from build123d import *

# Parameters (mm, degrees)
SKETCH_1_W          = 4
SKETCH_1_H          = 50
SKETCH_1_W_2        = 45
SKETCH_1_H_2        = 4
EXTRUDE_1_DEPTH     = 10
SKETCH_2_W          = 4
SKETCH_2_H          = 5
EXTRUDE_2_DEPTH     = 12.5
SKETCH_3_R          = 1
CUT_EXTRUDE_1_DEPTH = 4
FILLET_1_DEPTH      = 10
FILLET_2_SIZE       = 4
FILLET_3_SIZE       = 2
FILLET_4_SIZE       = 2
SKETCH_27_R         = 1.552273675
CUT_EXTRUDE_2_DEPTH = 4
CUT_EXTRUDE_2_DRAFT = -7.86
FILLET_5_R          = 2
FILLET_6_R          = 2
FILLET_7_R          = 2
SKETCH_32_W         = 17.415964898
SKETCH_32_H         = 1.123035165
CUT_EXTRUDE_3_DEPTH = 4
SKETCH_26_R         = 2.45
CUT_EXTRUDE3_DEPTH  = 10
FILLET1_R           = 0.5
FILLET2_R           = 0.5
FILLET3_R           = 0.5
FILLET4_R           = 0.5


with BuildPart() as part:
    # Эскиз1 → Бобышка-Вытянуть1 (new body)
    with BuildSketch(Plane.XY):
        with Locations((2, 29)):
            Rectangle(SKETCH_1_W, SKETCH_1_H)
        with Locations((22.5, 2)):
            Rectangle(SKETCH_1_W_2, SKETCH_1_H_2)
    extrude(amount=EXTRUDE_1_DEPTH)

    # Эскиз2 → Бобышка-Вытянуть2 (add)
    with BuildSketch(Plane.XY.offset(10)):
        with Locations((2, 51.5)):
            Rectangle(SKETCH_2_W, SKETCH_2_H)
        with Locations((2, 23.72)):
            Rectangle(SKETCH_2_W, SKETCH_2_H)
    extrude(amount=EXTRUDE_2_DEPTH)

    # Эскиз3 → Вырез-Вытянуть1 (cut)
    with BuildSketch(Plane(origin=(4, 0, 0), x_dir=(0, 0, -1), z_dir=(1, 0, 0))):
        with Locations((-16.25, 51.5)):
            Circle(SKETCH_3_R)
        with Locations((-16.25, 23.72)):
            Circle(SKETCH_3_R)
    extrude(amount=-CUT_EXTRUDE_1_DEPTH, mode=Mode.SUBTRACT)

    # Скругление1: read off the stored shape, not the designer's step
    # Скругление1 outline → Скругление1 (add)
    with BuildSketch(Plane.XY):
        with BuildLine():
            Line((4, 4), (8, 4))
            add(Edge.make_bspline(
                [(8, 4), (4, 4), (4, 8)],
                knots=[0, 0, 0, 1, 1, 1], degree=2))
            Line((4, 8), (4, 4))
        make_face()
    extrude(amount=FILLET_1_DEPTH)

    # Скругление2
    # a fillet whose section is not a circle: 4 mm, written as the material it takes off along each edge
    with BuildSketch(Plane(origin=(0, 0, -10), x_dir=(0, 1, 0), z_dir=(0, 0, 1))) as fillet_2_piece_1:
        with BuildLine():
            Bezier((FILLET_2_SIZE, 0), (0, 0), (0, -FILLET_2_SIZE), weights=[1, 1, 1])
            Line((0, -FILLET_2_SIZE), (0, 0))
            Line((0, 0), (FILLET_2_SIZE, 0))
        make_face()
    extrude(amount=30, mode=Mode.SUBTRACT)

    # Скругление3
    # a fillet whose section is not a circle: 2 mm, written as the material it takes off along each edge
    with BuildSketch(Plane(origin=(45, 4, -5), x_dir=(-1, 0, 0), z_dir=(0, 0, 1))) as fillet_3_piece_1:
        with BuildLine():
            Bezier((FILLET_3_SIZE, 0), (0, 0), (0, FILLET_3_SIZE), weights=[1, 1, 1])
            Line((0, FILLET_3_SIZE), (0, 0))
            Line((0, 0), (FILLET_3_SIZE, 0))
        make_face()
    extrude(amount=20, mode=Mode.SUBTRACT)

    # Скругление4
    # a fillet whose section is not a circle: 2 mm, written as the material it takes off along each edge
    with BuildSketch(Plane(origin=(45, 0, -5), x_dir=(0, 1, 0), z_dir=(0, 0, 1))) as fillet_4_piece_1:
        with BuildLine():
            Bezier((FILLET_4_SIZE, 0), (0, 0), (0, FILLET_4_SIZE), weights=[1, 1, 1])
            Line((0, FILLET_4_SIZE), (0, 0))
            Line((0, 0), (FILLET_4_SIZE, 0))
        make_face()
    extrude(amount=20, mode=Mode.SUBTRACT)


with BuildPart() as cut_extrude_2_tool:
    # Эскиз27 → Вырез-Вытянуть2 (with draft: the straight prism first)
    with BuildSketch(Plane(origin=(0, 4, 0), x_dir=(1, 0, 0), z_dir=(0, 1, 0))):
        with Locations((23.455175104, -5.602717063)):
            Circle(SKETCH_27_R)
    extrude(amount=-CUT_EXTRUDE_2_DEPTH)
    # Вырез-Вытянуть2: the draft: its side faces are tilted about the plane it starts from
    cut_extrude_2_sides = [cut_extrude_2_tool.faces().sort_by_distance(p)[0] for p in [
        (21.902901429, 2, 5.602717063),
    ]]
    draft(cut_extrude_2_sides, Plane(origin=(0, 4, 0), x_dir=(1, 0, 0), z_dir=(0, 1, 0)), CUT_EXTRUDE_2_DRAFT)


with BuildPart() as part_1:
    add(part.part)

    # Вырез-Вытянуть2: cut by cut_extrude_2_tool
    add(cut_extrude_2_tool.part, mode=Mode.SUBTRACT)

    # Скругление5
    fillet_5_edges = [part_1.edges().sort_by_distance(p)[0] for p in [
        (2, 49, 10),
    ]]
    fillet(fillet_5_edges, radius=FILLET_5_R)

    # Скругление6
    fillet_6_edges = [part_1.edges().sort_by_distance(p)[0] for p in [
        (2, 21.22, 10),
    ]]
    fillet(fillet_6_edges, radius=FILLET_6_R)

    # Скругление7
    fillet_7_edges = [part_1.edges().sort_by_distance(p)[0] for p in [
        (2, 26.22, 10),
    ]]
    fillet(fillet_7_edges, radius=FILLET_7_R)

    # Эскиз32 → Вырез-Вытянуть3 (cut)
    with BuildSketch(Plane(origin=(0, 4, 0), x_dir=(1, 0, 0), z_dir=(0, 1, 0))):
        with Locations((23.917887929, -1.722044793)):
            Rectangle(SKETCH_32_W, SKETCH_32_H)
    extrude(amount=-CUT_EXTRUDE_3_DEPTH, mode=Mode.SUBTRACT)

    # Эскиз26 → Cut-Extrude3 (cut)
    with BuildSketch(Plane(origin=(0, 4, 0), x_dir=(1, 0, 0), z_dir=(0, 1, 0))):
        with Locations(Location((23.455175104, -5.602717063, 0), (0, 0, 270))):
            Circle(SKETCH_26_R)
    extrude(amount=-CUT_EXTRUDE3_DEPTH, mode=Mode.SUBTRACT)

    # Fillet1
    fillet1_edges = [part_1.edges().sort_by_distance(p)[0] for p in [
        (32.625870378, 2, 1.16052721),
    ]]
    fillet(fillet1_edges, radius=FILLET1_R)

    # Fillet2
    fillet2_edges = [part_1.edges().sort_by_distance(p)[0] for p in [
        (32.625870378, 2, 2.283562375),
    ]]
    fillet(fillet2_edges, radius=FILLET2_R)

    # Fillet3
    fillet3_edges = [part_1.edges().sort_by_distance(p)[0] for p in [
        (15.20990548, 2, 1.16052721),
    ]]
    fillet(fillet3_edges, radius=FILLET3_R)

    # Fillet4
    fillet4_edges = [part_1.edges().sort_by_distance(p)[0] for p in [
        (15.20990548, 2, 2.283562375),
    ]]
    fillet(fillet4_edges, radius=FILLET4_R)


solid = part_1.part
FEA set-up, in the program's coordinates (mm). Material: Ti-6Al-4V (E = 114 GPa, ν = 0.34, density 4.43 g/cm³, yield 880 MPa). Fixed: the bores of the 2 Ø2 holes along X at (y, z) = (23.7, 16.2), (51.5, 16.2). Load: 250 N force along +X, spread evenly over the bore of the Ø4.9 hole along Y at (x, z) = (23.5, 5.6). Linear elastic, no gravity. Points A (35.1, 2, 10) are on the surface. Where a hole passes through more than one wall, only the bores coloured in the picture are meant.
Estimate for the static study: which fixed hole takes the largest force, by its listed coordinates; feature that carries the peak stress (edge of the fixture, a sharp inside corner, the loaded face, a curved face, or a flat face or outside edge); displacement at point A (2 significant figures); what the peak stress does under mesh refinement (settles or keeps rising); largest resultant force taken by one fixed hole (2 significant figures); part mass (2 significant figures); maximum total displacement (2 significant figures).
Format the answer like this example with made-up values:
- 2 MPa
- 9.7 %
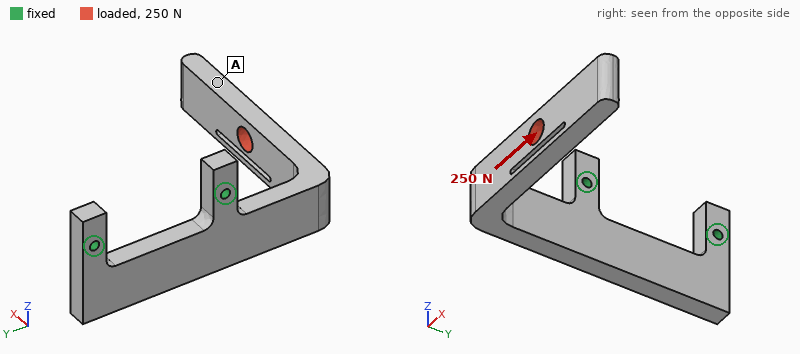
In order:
- (23.7, 16.2)
- edge of the fixture
- 0.58 mm
- keeps rising
- 380 N
- 18 g
- 0.74 mm
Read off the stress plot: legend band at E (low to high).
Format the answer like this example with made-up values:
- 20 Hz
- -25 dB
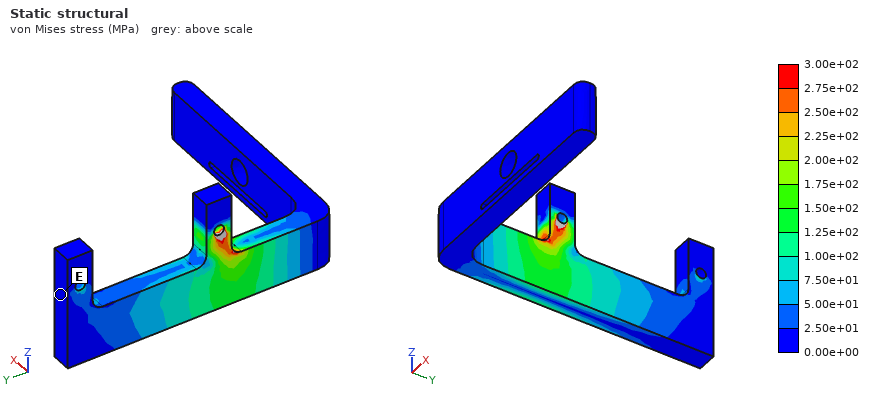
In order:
- 0.00e+00 to 2.50e+01 MPa
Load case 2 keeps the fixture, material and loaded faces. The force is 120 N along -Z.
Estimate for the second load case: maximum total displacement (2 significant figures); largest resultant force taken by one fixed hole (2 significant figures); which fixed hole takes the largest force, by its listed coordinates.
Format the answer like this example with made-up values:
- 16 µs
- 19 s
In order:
- 0.54 mm
- 220 N
- (23.7, 16.2)
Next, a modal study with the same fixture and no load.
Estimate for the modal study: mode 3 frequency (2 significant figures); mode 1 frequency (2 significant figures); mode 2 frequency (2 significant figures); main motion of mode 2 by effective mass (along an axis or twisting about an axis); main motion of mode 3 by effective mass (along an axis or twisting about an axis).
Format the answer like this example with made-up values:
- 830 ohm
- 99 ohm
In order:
- 2700 Hz
- 910 Hz
- 1100 Hz
- along Z
- along X
